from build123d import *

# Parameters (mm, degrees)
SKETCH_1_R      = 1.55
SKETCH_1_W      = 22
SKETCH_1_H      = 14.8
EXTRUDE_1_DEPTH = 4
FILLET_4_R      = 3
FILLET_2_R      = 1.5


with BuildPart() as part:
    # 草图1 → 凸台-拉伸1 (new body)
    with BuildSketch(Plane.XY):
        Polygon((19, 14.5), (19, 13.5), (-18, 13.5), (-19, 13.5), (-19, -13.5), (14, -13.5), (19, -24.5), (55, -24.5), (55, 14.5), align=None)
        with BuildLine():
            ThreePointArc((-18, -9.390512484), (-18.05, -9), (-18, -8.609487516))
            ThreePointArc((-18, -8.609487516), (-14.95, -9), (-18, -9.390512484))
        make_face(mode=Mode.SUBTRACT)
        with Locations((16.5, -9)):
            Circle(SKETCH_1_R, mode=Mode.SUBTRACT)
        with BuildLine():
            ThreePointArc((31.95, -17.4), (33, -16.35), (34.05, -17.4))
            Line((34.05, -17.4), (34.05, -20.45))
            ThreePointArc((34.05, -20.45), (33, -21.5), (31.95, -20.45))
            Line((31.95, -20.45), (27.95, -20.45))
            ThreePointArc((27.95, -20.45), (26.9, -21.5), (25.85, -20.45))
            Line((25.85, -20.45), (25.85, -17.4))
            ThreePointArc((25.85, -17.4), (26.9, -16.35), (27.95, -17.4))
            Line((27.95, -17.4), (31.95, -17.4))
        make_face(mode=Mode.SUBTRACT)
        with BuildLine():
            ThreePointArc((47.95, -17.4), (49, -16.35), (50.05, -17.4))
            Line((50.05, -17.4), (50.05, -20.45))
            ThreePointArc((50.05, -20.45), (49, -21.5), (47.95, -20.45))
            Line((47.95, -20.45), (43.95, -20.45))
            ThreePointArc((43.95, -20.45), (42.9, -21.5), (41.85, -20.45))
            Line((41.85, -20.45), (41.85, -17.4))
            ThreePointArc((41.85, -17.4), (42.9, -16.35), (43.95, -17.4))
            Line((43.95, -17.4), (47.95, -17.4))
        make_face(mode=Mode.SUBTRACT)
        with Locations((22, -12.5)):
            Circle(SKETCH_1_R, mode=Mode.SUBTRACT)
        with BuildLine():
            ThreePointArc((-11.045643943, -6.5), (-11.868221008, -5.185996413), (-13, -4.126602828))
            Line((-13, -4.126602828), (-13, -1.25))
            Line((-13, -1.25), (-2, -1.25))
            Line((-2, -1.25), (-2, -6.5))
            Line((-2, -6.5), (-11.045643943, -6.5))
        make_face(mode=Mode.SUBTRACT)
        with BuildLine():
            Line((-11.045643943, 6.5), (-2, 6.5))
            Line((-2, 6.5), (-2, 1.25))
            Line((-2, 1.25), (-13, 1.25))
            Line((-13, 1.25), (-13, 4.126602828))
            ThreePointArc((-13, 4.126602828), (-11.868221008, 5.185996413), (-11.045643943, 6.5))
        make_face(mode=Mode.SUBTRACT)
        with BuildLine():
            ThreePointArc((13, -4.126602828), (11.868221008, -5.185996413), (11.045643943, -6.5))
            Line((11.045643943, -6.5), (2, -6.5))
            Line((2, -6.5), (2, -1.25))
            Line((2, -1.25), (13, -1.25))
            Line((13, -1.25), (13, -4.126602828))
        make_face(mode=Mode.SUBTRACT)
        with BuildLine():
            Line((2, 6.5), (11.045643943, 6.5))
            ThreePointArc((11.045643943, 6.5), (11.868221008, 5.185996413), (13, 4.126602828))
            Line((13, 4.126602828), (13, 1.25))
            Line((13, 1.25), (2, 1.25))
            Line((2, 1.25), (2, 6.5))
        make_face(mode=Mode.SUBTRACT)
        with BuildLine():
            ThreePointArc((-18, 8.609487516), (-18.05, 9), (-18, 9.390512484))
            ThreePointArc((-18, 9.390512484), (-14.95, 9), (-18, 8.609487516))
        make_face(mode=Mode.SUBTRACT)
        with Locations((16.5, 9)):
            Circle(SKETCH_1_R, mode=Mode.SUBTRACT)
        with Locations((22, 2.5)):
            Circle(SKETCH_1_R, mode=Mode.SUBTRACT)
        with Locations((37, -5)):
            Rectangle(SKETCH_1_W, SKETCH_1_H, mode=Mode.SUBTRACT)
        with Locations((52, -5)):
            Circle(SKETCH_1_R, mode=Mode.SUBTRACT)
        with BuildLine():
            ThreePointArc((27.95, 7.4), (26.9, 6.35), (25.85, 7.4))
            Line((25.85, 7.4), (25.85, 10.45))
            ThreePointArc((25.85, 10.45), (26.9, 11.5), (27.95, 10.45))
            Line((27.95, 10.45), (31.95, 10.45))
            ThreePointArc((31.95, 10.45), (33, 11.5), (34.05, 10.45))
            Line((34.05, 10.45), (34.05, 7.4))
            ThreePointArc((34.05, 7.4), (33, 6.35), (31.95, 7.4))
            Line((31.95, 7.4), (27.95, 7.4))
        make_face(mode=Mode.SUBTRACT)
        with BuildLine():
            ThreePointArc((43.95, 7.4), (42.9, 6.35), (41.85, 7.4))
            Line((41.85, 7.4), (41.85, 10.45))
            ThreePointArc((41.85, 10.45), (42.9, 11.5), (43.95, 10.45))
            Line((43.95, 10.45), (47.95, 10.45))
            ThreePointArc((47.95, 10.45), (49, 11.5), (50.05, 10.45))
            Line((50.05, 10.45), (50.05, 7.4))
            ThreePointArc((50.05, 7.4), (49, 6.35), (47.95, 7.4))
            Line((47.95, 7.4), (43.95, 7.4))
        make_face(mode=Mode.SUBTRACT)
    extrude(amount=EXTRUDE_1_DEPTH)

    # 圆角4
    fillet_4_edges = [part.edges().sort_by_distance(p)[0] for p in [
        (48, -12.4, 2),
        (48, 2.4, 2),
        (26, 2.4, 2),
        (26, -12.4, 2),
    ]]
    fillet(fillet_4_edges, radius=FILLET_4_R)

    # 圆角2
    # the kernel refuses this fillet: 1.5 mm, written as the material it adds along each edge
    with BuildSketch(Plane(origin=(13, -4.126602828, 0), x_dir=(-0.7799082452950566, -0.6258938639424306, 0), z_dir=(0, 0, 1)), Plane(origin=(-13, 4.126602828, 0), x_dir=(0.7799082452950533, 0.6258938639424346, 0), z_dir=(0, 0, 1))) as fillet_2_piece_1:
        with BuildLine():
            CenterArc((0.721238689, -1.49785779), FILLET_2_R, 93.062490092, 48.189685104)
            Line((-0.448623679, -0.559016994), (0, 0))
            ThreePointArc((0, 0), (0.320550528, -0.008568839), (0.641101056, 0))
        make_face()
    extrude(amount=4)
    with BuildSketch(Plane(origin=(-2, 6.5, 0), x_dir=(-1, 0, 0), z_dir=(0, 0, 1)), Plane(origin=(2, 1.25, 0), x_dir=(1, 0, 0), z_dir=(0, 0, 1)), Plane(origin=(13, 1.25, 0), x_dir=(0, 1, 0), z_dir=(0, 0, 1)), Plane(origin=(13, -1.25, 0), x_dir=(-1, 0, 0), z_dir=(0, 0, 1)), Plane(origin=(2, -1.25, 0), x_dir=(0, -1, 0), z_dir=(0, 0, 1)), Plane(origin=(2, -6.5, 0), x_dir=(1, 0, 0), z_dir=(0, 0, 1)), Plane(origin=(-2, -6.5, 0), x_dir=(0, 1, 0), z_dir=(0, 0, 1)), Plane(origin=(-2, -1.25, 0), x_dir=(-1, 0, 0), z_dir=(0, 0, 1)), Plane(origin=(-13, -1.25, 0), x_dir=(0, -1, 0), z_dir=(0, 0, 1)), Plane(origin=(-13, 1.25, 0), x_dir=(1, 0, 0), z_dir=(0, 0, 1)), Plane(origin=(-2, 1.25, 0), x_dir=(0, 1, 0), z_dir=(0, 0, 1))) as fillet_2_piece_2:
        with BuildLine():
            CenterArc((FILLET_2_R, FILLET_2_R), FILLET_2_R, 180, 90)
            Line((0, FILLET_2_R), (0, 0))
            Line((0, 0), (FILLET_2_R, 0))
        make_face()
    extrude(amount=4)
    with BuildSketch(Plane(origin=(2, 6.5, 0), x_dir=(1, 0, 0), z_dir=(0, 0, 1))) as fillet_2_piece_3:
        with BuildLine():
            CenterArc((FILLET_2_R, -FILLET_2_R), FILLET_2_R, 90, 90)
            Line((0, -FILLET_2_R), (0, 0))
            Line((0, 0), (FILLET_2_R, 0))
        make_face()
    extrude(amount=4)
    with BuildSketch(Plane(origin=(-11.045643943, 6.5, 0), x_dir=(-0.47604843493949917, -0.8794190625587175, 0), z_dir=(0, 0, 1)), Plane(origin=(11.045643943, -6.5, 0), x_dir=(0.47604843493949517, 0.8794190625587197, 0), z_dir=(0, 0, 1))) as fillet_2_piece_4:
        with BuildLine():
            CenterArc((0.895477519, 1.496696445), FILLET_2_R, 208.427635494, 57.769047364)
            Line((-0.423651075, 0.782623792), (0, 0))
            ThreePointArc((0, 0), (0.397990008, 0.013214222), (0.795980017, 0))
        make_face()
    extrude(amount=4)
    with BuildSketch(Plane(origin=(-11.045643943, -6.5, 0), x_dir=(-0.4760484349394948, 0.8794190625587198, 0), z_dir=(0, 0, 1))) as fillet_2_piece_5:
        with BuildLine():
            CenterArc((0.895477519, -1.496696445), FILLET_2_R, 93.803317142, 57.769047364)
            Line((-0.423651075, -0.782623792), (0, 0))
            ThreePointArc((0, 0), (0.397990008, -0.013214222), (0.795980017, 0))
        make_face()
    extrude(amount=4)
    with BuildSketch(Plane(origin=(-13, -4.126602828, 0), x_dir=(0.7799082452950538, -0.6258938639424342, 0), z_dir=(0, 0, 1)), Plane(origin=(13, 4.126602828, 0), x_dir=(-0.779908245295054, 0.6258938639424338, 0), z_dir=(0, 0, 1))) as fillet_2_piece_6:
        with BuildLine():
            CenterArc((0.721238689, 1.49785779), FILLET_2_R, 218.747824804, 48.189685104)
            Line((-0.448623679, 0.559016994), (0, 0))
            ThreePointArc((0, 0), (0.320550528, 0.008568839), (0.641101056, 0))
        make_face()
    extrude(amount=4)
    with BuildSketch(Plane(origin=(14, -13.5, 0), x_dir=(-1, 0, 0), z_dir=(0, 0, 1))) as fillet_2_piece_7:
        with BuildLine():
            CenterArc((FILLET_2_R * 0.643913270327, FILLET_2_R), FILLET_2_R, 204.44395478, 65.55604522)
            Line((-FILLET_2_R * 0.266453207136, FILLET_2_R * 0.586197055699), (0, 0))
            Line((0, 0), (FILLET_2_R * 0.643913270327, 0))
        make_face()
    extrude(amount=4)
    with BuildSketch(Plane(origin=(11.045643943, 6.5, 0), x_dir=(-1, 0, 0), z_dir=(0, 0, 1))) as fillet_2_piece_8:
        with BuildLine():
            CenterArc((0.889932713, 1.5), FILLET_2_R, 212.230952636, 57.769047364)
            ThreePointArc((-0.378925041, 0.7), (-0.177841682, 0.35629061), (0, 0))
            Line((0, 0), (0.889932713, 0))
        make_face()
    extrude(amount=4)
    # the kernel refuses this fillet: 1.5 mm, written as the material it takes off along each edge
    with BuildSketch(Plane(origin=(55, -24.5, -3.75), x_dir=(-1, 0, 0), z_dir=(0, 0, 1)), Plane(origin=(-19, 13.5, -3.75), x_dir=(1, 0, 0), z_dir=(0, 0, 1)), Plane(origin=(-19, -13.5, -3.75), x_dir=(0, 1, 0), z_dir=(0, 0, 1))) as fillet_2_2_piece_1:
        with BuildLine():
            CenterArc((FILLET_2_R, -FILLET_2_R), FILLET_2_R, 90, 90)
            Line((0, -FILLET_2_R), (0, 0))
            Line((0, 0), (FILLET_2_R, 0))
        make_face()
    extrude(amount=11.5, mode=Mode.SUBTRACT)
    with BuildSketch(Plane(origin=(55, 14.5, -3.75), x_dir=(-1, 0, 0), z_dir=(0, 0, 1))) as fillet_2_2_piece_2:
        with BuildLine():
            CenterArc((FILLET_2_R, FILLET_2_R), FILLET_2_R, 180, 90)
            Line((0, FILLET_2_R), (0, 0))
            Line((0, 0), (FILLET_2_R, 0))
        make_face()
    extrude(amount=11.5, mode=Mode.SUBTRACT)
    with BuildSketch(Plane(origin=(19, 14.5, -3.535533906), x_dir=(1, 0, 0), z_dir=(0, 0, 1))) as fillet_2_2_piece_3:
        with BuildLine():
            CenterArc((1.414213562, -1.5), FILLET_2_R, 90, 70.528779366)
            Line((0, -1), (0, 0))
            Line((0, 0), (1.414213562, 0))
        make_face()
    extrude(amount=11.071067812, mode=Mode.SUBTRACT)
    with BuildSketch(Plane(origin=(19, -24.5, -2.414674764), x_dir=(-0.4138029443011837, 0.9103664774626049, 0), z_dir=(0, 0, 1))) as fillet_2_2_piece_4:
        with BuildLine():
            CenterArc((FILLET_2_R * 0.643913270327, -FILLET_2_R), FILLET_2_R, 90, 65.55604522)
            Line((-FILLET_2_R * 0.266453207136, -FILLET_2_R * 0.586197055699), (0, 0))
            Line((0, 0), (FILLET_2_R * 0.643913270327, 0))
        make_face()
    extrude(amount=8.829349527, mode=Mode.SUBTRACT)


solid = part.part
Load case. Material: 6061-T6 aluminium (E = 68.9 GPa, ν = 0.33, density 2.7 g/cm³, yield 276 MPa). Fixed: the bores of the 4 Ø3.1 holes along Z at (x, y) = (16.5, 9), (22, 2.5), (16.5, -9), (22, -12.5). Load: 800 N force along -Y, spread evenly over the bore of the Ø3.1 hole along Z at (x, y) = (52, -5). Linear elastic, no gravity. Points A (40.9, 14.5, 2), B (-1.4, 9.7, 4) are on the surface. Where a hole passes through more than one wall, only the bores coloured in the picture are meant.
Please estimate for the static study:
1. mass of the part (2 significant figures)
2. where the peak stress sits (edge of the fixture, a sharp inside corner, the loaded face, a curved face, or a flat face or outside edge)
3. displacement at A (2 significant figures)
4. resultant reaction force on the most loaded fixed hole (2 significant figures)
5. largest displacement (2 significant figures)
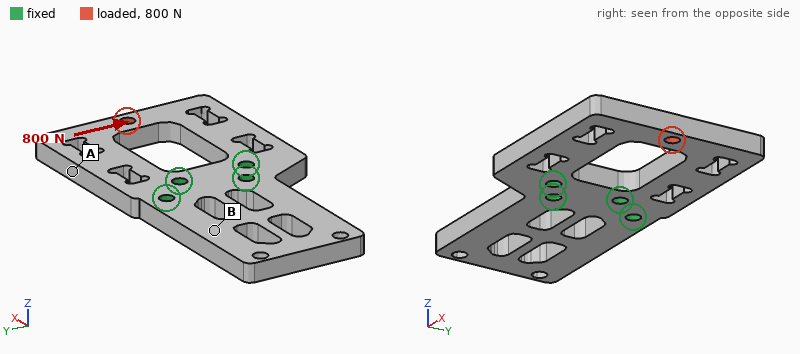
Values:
19 g
a curved face
56 µm
1.0 kN
98 µm
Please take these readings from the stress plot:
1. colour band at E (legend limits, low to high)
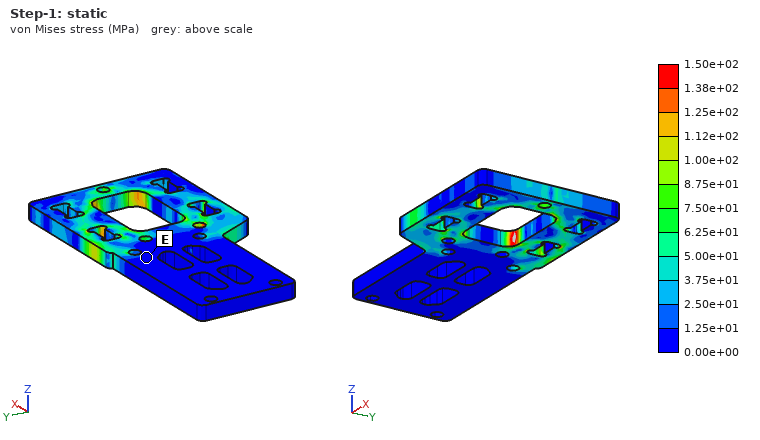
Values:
0.00e+00 to 1.25e+01 MPa
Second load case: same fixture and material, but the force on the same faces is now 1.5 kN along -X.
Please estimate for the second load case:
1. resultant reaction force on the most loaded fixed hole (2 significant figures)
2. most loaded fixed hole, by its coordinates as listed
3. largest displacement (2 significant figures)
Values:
840 N
(22, -12.5)
40 µm
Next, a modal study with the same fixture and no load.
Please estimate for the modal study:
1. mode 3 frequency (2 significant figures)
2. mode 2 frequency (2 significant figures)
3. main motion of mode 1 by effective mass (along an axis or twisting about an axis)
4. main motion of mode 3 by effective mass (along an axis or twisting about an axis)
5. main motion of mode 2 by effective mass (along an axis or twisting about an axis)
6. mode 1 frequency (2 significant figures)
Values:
4200 Hz
2500 Hz
along Z
twisting about X
along Z
2300 Hz
